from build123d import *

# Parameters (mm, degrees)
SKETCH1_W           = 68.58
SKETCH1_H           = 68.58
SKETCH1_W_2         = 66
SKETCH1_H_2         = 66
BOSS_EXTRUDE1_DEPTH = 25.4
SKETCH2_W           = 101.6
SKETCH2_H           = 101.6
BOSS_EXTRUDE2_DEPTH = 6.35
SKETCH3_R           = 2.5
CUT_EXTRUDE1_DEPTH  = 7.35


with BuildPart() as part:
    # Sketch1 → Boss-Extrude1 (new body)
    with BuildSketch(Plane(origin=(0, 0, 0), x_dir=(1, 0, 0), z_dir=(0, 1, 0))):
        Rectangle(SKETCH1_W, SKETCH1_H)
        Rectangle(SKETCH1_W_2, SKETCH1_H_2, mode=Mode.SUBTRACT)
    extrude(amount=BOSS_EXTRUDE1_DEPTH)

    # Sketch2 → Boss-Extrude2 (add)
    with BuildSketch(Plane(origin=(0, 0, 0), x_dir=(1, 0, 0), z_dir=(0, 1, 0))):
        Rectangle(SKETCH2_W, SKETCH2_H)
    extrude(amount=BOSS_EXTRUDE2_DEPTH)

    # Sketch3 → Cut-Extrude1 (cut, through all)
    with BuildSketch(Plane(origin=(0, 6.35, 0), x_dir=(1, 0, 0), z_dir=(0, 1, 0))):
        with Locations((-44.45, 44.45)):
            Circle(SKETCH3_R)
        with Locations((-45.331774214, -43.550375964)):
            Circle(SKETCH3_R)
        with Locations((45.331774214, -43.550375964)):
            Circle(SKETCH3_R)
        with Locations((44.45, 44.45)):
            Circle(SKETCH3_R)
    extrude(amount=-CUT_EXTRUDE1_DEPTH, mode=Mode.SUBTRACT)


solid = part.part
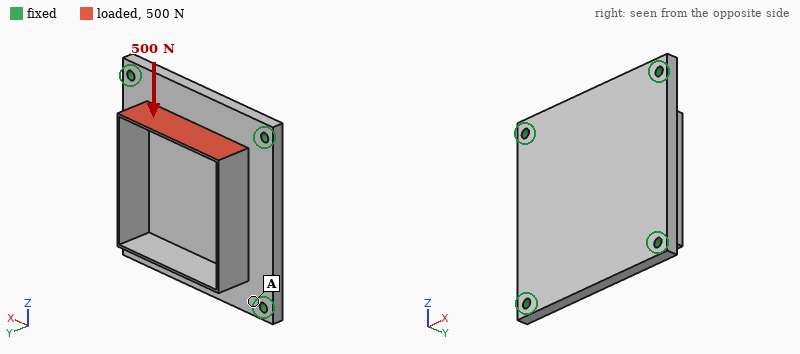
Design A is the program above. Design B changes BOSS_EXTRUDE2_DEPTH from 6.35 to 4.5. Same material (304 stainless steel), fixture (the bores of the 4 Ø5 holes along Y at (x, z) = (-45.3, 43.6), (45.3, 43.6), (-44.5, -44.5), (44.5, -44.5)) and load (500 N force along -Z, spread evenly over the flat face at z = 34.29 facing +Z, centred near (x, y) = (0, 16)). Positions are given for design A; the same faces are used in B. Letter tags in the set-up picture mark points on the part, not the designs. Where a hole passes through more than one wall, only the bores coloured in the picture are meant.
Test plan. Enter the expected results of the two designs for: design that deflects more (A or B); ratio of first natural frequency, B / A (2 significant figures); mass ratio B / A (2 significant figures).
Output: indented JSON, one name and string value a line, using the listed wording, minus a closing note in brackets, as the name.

{
  "design that deflects more": "B",
  "ratio of first natural frequency, B / A": "0.86",
  "mass ratio B / A": "0.74"
}
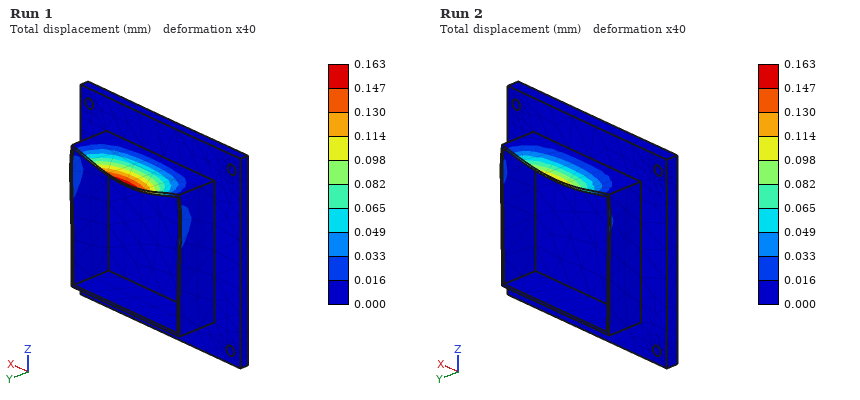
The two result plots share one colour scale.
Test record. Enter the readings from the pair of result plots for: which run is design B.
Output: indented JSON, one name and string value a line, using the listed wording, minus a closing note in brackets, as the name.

{
  "which run is design B": "Run 1"
}
